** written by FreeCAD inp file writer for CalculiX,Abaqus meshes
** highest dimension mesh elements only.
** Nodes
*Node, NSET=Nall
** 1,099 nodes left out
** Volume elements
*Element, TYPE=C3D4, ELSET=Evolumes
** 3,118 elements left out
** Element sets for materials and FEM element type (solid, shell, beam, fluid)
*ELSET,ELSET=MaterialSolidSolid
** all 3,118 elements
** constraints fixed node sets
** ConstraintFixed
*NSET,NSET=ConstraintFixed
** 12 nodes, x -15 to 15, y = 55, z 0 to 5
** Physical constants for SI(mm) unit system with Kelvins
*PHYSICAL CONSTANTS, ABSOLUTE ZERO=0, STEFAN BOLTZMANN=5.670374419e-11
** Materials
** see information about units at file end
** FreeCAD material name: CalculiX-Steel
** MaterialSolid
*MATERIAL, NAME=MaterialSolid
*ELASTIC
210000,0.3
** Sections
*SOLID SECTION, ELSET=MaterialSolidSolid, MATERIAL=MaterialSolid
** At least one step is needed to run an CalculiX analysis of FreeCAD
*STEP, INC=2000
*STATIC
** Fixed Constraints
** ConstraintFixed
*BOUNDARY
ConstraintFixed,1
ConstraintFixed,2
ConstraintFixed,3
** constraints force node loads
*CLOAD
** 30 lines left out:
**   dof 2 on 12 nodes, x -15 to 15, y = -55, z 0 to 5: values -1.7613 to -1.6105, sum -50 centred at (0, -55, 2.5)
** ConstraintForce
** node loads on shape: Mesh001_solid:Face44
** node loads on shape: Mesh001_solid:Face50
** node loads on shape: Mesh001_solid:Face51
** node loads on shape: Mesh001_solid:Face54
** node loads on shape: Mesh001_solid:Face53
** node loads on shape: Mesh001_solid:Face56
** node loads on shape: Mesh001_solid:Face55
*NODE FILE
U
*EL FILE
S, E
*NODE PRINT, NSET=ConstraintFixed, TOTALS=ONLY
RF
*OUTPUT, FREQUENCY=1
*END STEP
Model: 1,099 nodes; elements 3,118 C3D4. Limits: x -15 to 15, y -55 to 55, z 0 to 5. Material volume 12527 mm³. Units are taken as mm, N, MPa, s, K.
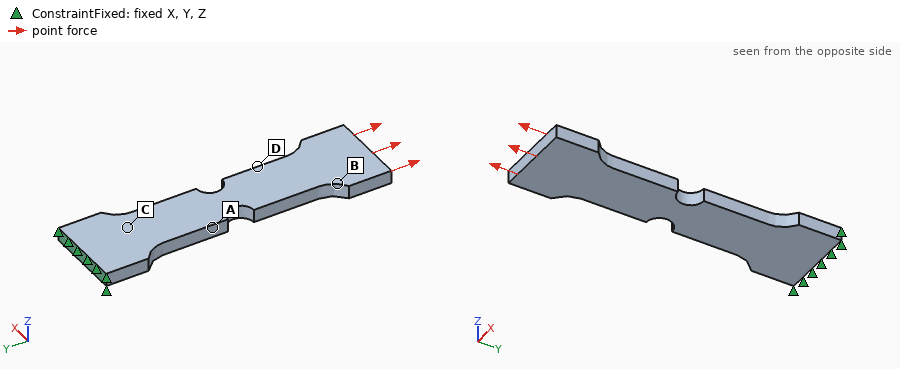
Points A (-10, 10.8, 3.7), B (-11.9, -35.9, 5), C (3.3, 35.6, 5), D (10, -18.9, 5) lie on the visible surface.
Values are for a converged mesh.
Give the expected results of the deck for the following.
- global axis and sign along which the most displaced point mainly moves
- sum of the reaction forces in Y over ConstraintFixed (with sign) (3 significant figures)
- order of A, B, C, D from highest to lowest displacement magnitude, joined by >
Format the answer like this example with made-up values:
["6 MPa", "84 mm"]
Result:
["-Y", "50.0 N", "B > D > A > C"]
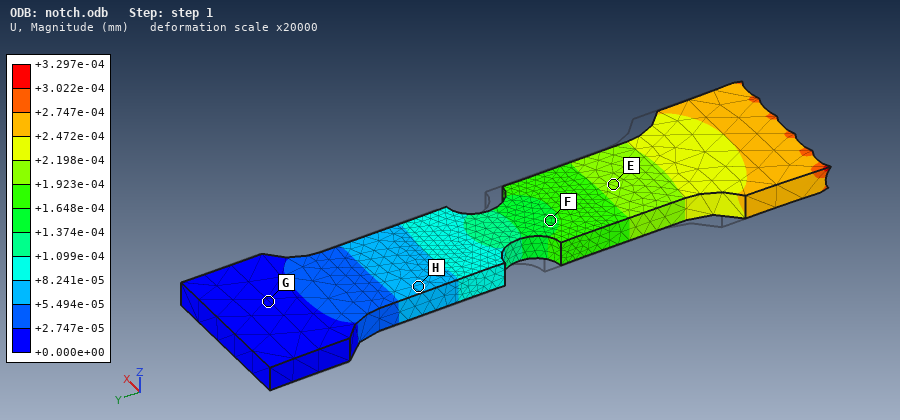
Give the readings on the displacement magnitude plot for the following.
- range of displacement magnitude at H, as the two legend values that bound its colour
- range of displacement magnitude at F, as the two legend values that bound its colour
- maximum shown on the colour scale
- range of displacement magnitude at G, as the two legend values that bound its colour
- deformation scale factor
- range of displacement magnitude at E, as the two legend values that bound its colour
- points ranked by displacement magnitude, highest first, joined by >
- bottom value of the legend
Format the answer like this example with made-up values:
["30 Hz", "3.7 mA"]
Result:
["+5.494e-05 to +8.241e-05 mm", "+1.374e-04 to +1.648e-04 mm", "+3.297e-04 mm", "+0.000e+00 to +2.747e-05 mm", "20000", "+1.923e-04 to +2.198e-04 mm", "E > F > H > G", "+0.000e+00 mm"]
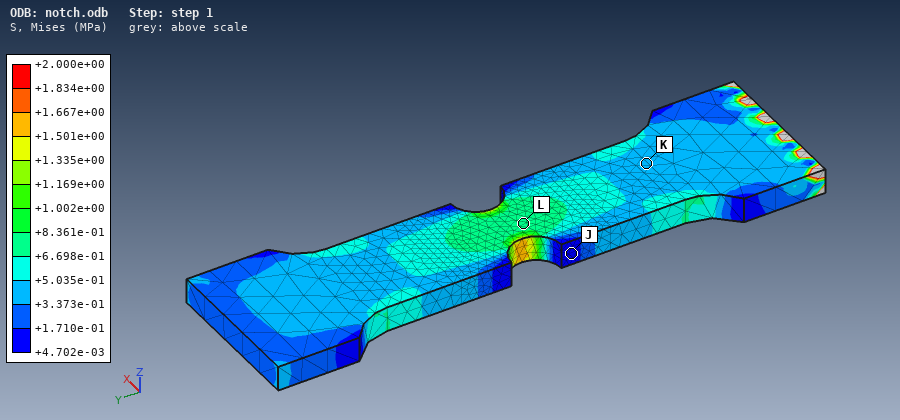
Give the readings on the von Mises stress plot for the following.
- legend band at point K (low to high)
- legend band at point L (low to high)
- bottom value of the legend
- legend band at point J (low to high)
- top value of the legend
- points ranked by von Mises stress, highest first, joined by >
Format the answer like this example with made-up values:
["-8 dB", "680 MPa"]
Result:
["+3.373e-01 to +5.035e-01 MPa", "+6.698e-01 to +8.361e-01 MPa", "+4.702e-03 MPa", "+4.702e-03 to +1.710e-01 MPa", "+2.000e+00 MPa", "L > K > J"]
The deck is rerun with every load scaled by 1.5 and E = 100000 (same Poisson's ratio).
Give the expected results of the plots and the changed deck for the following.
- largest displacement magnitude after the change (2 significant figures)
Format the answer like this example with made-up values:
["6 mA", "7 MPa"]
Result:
["0.0010 mm"]
